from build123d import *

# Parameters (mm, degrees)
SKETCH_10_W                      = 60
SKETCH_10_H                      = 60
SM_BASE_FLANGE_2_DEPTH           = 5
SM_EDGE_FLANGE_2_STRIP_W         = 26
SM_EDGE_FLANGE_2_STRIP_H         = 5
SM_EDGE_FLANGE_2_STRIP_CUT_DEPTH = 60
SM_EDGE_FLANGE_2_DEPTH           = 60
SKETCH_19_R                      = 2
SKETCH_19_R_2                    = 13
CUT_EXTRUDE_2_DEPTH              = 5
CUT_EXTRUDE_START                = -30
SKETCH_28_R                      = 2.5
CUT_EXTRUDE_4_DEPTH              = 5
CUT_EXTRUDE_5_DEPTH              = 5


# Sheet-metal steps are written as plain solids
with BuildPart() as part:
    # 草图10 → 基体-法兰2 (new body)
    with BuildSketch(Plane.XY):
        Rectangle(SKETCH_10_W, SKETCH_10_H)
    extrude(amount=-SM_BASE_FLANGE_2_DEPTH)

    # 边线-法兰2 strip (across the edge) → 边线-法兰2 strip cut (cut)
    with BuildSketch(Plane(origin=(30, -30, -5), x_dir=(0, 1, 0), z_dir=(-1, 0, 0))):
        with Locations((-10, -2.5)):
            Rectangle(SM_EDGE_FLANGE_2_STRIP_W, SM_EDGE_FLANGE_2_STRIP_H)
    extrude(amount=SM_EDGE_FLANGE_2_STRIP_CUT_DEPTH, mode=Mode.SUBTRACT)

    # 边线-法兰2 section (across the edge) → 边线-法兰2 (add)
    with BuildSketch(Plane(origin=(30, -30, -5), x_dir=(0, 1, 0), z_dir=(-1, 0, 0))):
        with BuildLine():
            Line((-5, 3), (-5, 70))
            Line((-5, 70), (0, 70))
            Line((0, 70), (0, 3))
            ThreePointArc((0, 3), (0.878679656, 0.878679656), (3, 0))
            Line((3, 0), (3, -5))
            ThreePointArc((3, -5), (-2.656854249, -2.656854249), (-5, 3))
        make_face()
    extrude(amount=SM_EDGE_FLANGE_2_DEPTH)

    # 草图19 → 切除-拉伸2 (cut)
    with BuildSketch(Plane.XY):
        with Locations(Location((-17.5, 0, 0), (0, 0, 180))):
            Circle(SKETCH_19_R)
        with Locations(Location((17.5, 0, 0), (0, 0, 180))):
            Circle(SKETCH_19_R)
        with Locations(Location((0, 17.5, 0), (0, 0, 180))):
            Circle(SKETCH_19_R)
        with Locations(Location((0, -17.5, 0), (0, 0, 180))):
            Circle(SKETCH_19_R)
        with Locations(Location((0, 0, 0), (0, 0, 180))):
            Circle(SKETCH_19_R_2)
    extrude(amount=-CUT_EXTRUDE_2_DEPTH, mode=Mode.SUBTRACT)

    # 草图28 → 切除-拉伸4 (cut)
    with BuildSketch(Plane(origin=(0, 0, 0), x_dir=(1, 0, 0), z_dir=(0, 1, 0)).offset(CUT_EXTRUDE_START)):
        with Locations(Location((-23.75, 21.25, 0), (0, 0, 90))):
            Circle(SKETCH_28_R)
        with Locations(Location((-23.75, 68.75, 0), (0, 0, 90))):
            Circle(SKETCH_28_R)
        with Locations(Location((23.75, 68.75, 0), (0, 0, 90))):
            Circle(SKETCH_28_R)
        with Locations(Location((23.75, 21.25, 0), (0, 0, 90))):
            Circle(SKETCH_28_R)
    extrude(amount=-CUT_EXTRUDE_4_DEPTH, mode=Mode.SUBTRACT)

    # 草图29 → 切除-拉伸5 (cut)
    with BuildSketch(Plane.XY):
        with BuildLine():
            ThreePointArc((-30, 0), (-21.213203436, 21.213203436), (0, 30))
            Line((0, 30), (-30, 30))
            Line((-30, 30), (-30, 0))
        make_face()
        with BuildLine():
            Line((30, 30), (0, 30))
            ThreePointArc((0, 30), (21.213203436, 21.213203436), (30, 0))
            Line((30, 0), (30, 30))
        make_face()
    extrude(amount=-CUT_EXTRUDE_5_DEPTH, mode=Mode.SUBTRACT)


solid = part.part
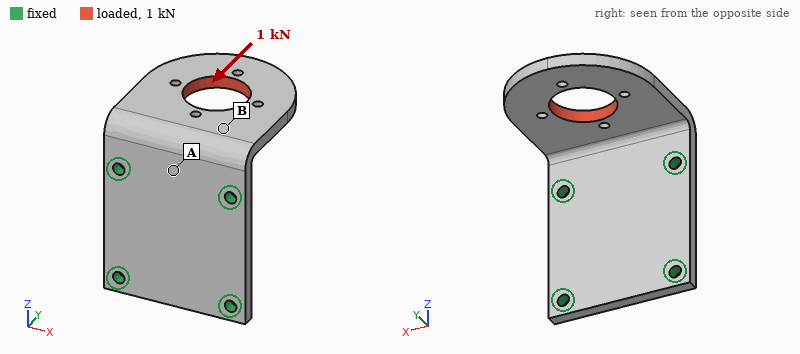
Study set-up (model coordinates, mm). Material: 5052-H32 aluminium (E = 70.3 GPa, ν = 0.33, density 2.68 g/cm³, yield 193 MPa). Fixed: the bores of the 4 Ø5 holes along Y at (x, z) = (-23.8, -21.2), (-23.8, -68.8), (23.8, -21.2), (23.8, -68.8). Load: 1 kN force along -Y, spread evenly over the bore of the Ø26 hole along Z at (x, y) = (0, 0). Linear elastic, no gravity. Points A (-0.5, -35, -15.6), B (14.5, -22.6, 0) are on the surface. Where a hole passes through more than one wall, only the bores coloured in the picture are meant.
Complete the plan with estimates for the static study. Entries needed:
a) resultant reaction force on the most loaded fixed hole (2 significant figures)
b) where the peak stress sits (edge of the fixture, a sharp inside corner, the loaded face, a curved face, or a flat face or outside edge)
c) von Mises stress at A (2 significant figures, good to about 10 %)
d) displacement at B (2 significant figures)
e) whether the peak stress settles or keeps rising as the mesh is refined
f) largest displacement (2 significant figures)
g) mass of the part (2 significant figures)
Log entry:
550 N
edge of the fixture
26 MPa
0.085 mm
keeps rising
0.28 mm
93 g
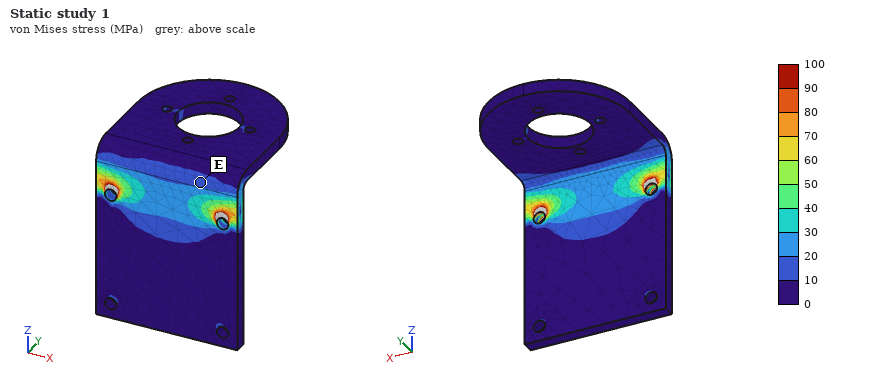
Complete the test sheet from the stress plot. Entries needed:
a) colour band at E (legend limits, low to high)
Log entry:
10 to 20 MPa
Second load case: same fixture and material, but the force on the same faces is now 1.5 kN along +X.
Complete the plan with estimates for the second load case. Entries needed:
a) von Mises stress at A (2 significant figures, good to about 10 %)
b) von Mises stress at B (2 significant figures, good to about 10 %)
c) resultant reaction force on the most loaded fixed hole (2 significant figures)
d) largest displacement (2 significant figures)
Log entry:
23 MPa
23 MPa
1.4 kN
0.23 mm
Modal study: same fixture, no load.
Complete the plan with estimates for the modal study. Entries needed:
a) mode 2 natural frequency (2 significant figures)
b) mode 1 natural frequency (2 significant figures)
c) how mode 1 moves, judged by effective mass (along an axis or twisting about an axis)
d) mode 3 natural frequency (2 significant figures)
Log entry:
2200 Hz
890 Hz
along Z
3400 Hz
